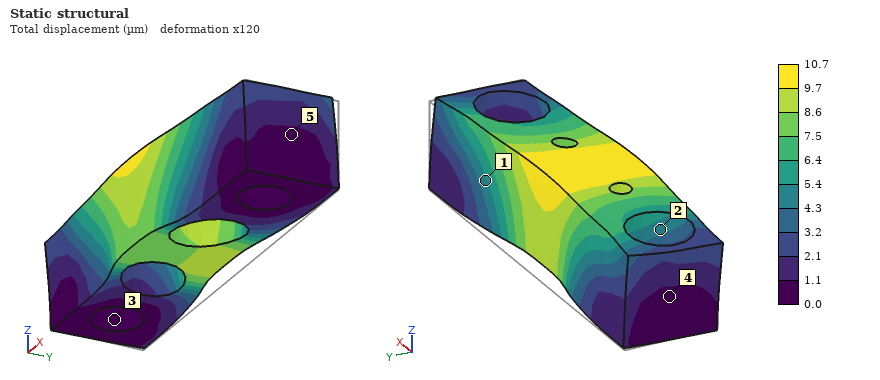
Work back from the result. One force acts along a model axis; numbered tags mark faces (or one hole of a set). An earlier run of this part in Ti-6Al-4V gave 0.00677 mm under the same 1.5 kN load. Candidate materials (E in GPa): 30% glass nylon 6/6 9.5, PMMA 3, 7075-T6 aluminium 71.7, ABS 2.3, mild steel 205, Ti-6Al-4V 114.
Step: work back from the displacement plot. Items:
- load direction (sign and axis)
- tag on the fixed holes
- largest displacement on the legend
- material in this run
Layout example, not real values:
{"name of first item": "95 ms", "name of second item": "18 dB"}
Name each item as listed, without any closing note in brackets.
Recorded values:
{"load direction": "-Y", "tag on the fixed holes": "3", "largest displacement on the legend": "10.7 µm", "material in this run": "7075-T6 aluminium"}
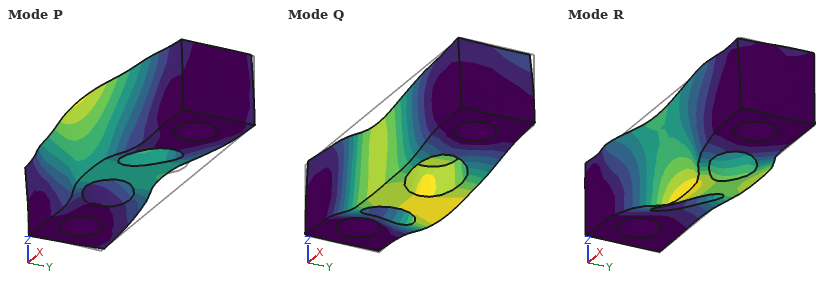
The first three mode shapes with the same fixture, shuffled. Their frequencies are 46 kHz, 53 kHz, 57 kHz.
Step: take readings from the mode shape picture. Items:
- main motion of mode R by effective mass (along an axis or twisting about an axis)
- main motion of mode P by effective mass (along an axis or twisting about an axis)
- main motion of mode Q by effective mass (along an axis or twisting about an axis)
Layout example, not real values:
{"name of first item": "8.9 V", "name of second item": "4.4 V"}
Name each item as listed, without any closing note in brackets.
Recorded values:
{"main motion of mode R by effective mass": "twisting about X", "main motion of mode P by effective mass": "along Y", "main motion of mode Q by effective mass": "along Z"}
